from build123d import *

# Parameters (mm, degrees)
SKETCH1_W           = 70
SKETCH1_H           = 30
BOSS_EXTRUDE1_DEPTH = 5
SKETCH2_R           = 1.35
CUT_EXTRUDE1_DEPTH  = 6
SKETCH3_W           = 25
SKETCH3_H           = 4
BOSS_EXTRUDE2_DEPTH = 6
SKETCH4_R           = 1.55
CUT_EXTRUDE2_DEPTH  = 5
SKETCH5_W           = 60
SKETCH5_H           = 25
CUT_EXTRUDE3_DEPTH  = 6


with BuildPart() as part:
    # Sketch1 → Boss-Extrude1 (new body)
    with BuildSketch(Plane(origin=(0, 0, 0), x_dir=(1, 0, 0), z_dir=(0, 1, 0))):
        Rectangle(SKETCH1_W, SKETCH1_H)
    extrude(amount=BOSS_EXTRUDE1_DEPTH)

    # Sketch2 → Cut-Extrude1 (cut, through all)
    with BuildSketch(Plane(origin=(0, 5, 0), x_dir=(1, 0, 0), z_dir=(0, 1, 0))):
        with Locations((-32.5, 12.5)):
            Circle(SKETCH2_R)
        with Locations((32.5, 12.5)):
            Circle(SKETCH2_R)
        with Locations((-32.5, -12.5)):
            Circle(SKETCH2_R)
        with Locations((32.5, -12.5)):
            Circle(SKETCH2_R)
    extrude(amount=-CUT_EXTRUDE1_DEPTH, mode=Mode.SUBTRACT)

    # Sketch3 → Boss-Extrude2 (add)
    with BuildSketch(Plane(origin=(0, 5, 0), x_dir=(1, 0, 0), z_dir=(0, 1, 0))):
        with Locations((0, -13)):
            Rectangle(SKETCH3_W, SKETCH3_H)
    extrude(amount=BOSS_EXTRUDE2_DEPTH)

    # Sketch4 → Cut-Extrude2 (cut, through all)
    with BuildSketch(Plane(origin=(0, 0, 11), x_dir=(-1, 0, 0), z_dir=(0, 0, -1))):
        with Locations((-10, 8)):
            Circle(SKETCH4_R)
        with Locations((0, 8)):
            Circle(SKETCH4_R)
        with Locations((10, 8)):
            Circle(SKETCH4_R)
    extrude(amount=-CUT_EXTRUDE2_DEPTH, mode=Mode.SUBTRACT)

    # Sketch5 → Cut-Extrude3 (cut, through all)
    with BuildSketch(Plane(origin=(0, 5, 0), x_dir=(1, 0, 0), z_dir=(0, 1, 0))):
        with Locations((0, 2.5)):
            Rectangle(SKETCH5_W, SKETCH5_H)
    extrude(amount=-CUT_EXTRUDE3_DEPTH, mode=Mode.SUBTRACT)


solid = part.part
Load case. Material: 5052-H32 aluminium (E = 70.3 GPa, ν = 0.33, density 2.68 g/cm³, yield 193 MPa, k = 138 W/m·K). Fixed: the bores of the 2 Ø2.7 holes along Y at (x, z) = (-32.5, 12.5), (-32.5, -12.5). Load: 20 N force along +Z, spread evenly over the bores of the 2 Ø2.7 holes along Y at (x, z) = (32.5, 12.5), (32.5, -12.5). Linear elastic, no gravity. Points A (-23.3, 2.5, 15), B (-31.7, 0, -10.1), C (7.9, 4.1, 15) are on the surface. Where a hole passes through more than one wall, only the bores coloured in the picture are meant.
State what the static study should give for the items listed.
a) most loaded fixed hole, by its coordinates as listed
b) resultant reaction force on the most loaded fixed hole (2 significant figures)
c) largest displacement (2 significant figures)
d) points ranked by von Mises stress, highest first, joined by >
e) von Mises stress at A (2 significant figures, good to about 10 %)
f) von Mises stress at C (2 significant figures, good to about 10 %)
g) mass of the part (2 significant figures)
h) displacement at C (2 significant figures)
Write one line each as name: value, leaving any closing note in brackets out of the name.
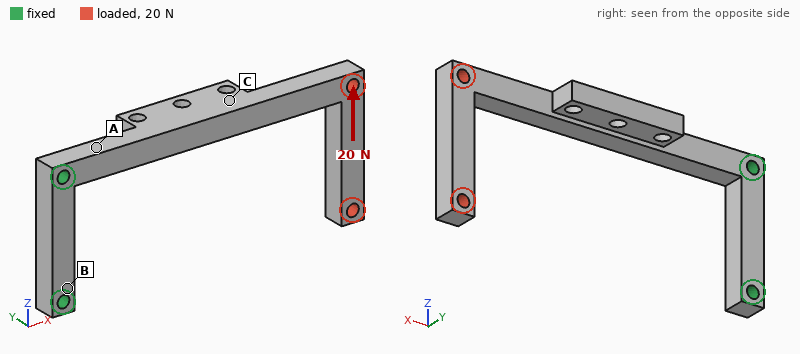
most loaded fixed hole, by its coordinates as listed: (-32.5, -12.5)
resultant reaction force on the most loaded fixed hole: 21 N
largest displacement: 0.56 mm
points ranked by von Mises stress, highest first, joined by >: A > C > B
von Mises stress at A: 54 MPa
von Mises stress at C: 17 MPa
mass of the part: 9.1 g
displacement at C: 0.22 mm
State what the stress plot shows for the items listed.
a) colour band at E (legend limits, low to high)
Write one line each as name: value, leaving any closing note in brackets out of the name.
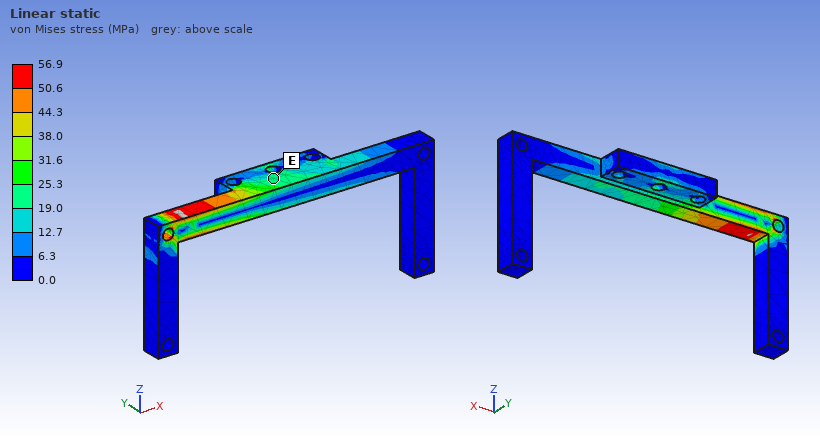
colour band at E: 19.0 to 25.3 MPa
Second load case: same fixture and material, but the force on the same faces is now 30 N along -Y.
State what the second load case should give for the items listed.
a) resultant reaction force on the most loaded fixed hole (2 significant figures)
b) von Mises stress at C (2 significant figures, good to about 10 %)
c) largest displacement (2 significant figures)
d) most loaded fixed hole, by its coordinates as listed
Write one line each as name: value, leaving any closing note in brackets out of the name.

resultant reaction force on the most loaded fixed hole: 33 N
von Mises stress at C: 17 MPa
largest displacement: 0.86 mm
most loaded fixed hole, by its coordinates as listed: (-32.5, 12.5)
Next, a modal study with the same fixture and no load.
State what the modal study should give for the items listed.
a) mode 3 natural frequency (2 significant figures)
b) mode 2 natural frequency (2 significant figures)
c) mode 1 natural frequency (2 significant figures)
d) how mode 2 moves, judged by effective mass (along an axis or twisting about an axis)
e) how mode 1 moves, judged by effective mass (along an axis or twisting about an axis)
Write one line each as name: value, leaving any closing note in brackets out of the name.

mode 3 natural frequency: 2100 Hz
mode 2 natural frequency: 640 Hz
mode 1 natural frequency: 590 Hz
how mode 2 moves, judged by effective mass: along Y
how mode 1 moves, judged by effective mass: along Z
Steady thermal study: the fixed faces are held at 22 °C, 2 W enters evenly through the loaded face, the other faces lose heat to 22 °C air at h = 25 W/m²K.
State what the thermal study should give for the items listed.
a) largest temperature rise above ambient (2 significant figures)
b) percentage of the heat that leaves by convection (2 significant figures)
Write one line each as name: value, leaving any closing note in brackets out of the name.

largest temperature rise above ambient: 28 K
percentage of the heat that leaves by convection: 39 %
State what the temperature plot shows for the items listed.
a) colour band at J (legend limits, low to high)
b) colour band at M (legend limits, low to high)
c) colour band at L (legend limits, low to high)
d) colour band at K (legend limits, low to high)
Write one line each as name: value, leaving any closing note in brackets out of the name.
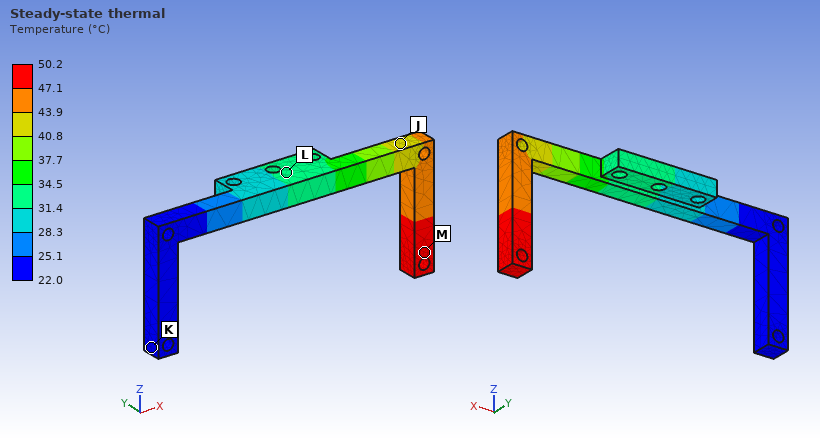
colour band at J: 40.8 to 43.9 °C
colour band at M: 47.1 to 50.2 °C
colour band at L: 31.4 to 34.5 °C
colour band at K: 22.0 to 25.1 °C
